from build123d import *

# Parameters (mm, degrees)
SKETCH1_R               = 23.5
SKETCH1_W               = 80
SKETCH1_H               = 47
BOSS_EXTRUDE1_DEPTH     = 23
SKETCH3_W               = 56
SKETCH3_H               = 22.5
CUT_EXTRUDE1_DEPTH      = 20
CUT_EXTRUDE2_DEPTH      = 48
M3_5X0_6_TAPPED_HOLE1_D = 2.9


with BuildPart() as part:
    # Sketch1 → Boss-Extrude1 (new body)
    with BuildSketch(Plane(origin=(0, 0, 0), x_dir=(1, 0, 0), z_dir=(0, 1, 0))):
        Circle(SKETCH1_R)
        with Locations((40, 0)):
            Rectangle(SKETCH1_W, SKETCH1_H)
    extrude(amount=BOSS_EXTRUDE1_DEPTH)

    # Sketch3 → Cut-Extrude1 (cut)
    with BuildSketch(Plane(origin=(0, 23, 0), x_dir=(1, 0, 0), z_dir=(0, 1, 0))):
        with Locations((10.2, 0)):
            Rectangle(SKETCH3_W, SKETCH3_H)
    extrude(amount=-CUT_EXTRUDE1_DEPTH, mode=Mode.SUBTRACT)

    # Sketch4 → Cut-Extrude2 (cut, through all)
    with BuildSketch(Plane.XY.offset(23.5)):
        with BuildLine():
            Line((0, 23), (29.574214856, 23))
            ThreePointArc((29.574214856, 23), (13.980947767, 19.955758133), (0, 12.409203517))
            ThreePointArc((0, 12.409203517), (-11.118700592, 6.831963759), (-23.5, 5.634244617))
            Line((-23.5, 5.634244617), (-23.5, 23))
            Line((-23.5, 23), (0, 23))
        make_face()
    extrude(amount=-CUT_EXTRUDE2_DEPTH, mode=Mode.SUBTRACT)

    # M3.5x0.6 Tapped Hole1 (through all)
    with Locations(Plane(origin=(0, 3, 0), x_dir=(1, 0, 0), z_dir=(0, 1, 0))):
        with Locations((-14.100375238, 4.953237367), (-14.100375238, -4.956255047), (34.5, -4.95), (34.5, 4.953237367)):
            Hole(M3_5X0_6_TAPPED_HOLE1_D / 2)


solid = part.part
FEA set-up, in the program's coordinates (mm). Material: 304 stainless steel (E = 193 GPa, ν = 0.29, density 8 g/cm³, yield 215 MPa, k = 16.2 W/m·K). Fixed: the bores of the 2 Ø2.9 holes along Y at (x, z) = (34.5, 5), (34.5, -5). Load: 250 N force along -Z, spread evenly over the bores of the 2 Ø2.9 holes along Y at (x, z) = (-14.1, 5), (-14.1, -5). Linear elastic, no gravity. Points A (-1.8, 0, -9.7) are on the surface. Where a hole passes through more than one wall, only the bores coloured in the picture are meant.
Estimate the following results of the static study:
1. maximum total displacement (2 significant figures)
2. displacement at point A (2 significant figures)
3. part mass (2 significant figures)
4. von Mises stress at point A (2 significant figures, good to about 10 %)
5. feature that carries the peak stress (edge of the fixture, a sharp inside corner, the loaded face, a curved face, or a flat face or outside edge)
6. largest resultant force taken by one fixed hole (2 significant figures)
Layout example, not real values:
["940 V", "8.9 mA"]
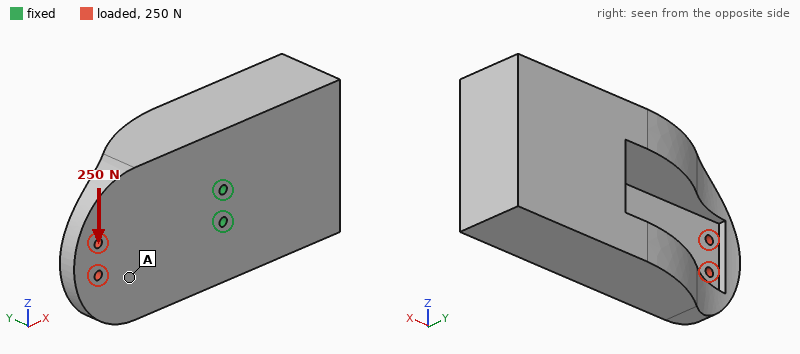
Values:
["13 µm", "8.1 µm", "570 g", "3.3 MPa", "edge of the fixture", "1.0 kN"]
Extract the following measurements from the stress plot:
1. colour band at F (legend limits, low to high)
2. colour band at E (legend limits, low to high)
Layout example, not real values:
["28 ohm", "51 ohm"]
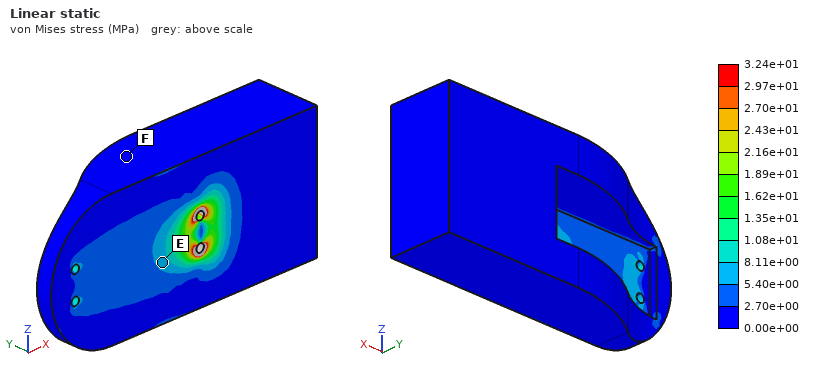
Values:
["0.00e+00 to 2.70e+00 MPa", "5.40e+00 to 8.11e+00 MPa"]
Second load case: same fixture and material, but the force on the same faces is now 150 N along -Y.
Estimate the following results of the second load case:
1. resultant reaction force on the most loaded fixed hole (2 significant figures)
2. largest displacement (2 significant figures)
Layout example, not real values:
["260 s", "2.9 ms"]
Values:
["83 N", "79 µm"]
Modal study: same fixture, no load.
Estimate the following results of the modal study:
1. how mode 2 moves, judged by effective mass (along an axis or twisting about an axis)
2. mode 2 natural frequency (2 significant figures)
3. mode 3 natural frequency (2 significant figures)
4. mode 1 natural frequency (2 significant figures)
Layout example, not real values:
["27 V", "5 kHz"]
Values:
["along Z", "1700 Hz", "1900 Hz", "570 Hz"]
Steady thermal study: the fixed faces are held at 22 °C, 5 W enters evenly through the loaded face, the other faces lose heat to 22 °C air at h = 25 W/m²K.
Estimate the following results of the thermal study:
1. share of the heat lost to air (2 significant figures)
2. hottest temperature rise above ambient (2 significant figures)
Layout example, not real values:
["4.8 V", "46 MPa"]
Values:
["74 %", "50 K"]
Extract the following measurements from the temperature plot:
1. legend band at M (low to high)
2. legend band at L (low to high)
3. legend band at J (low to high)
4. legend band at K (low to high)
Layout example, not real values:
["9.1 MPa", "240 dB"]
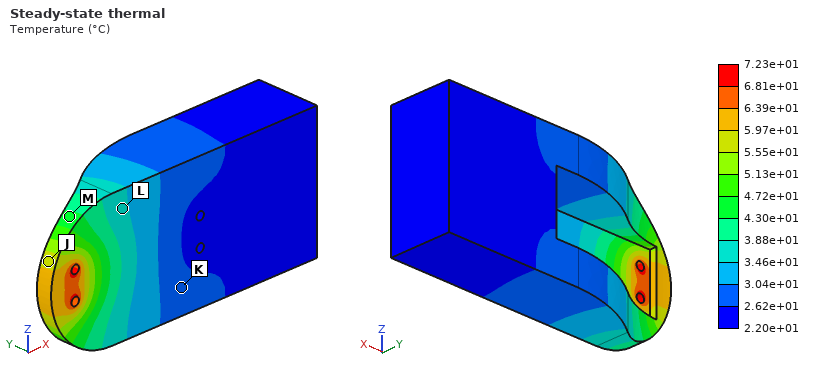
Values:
["4.30e+01 to 4.72e+01 °C", "3.46e+01 to 3.88e+01 °C", "5.55e+01 to 5.97e+01 °C", "2.62e+01 to 3.04e+01 °C"]
